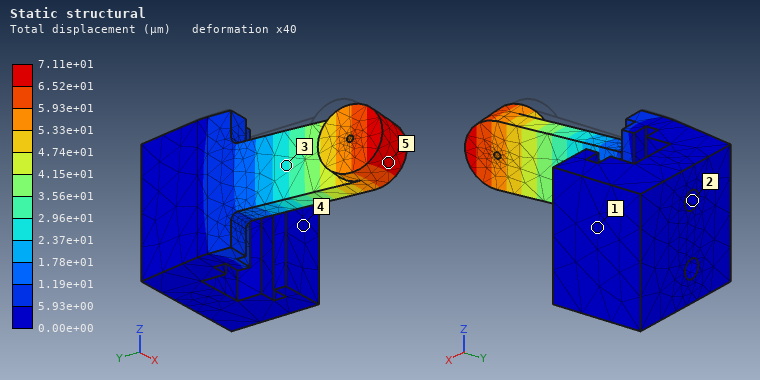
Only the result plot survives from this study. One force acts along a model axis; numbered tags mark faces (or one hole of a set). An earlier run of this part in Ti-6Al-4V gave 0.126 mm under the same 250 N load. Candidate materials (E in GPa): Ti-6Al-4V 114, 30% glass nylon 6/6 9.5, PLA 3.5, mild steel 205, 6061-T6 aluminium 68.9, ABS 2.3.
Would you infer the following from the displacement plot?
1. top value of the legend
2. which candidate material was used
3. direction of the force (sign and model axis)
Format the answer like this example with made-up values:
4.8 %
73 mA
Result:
7.11e+01 µm
mild steel
+X
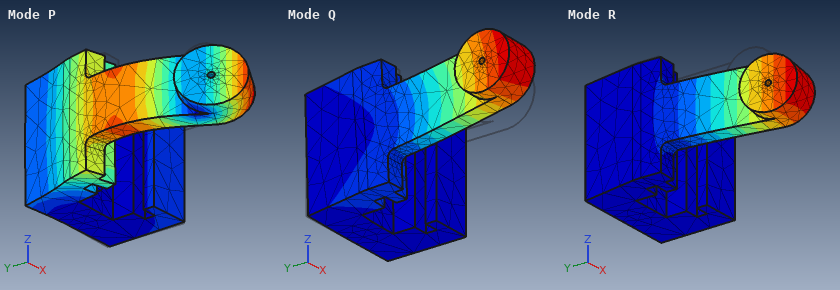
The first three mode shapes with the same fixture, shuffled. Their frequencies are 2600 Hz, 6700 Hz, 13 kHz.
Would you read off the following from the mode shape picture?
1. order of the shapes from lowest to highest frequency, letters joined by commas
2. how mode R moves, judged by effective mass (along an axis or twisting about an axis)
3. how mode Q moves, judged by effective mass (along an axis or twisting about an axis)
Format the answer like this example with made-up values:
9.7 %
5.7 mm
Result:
R, Q, P
along X
along Z
